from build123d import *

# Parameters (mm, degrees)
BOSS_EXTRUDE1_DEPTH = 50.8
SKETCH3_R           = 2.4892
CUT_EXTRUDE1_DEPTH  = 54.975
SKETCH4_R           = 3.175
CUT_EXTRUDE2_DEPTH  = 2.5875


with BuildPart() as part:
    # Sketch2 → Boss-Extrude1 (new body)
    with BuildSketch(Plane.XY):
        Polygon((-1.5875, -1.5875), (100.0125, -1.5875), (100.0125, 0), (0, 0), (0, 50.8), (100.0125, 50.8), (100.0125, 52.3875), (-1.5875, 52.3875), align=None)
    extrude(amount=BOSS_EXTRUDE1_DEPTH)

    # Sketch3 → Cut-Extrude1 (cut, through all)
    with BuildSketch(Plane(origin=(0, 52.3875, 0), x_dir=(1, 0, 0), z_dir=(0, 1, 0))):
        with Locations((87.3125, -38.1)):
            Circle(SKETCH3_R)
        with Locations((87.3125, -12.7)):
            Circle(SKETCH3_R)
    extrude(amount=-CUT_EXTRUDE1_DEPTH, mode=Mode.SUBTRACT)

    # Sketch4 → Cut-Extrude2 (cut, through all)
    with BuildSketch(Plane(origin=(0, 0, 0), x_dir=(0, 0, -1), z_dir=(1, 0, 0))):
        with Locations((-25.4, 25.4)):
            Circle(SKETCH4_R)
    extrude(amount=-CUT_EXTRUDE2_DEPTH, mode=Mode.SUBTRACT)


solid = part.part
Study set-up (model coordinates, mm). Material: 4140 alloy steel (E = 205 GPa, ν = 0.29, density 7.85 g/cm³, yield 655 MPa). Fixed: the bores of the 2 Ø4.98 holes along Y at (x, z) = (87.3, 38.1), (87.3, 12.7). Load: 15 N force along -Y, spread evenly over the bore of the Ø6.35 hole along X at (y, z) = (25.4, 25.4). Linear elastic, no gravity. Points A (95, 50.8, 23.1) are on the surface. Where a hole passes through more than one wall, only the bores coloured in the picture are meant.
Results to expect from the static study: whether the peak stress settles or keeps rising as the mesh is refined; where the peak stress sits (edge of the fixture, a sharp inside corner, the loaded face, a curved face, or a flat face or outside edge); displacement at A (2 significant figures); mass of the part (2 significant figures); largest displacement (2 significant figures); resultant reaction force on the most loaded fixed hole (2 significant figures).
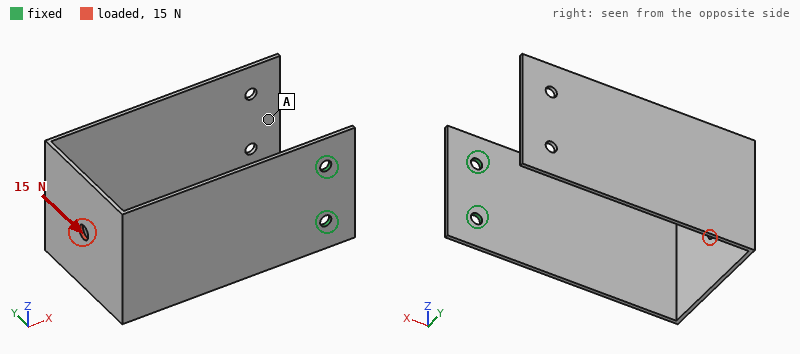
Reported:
keeps rising
edge of the fixture
1.0 mm
160 g
1.3 mm
7.5 N
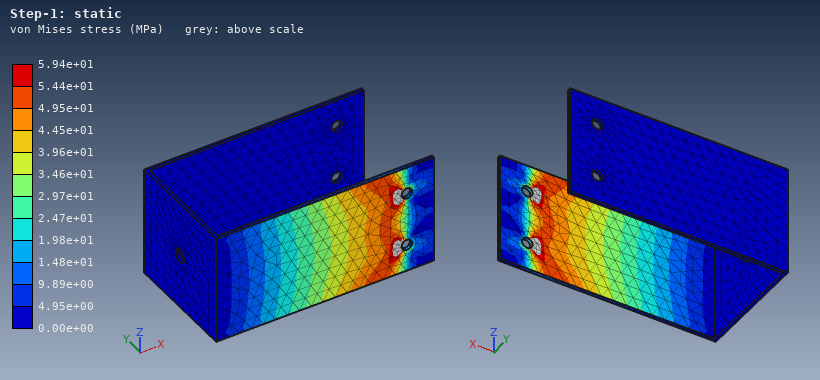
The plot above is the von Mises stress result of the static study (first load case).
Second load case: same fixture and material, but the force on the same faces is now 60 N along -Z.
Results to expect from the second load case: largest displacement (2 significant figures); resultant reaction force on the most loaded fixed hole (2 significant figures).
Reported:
1.4 mm
190 N
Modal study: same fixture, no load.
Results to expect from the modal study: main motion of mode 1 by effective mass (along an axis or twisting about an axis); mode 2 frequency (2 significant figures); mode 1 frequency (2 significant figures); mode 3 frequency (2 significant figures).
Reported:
along X
74 Hz
49 Hz
75 Hz
